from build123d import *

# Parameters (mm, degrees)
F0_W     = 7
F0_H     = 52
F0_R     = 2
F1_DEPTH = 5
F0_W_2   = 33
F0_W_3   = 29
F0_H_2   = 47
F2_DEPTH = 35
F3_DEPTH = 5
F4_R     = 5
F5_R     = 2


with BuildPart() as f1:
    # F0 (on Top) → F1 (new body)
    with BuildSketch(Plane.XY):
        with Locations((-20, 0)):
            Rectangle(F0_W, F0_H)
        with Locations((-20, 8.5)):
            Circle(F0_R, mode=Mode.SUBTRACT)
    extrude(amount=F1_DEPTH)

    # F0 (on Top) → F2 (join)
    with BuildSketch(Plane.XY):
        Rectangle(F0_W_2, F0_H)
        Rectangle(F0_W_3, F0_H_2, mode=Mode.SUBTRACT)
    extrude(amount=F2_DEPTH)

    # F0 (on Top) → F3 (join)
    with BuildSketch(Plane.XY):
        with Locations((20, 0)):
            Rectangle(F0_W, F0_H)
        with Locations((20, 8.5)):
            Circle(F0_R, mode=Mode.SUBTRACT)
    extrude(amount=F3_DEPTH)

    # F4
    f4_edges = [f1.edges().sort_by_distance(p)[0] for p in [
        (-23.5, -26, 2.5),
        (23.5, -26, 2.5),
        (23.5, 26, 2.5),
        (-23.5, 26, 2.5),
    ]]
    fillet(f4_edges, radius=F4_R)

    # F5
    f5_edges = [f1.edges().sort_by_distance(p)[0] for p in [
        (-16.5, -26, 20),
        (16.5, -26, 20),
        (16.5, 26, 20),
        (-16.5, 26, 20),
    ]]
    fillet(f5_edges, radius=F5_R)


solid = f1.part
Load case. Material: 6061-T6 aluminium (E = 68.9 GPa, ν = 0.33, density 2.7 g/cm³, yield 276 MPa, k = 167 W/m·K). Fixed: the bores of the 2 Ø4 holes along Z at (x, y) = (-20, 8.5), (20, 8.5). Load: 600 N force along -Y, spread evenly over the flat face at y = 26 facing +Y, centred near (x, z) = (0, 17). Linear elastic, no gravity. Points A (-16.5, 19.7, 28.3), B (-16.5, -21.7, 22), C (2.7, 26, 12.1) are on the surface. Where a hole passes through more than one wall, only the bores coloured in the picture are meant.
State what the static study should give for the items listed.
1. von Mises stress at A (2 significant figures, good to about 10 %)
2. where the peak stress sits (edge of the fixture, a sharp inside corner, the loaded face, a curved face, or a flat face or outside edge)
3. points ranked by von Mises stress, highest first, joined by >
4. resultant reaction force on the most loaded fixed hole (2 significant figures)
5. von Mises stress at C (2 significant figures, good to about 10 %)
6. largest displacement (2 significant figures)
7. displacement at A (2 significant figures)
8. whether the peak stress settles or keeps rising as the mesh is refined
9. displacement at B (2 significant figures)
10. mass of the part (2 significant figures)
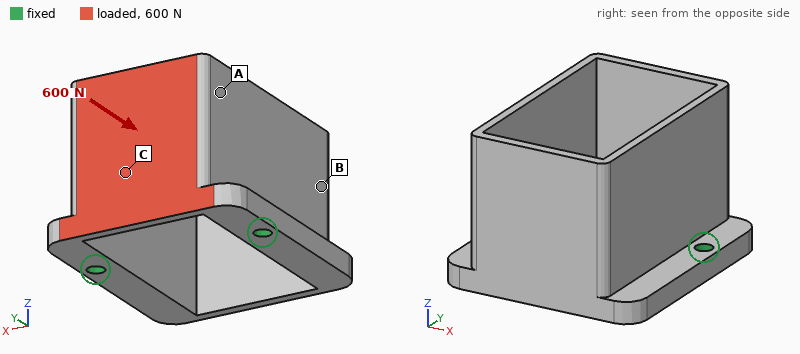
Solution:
18 MPa
edge of the fixture
C > A > B
320 N
28 MPa
97 µm
40 µm
keeps rising
48 µm
42 g
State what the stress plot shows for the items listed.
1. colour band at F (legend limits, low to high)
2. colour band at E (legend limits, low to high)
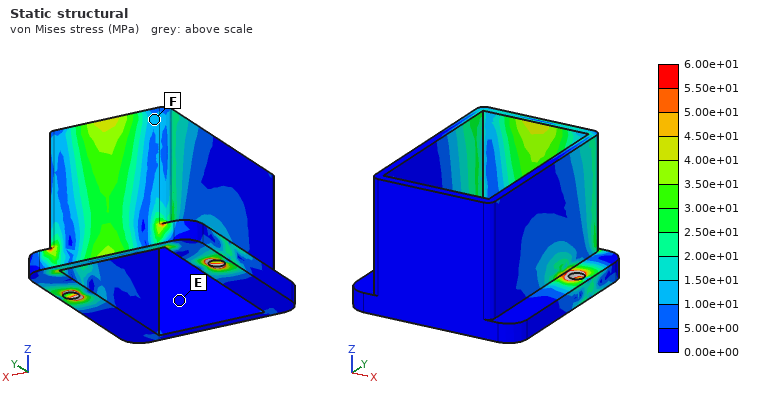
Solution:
1.00e+01 to 1.50e+01 MPa
0.00e+00 to 5.00e+00 MPa
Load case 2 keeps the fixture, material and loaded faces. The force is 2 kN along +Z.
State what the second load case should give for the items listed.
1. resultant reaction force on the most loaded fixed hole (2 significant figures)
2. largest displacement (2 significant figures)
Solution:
1.0 kN
0.24 mm
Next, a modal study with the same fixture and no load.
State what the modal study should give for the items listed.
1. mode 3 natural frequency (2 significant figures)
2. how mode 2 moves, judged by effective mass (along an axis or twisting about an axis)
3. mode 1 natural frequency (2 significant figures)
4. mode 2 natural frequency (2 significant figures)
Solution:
4200 Hz
along X
2400 Hz
2700 Hz
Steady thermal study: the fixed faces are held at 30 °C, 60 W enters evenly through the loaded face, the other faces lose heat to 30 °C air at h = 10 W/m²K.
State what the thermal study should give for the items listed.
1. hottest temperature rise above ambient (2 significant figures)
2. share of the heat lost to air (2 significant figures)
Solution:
67 K
4.7 %
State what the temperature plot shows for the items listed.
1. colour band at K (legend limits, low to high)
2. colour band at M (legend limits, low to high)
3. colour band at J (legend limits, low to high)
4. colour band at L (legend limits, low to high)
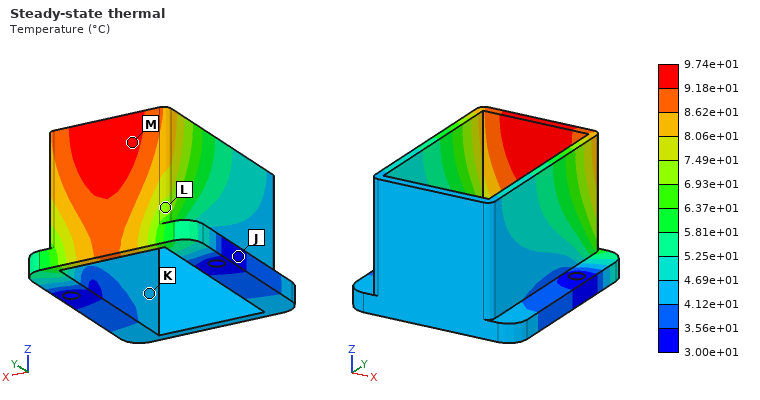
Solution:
4.12e+01 to 4.69e+01 °C
9.18e+01 to 9.74e+01 °C
3.00e+01 to 3.56e+01 °C
6.93e+01 to 7.49e+01 °C
